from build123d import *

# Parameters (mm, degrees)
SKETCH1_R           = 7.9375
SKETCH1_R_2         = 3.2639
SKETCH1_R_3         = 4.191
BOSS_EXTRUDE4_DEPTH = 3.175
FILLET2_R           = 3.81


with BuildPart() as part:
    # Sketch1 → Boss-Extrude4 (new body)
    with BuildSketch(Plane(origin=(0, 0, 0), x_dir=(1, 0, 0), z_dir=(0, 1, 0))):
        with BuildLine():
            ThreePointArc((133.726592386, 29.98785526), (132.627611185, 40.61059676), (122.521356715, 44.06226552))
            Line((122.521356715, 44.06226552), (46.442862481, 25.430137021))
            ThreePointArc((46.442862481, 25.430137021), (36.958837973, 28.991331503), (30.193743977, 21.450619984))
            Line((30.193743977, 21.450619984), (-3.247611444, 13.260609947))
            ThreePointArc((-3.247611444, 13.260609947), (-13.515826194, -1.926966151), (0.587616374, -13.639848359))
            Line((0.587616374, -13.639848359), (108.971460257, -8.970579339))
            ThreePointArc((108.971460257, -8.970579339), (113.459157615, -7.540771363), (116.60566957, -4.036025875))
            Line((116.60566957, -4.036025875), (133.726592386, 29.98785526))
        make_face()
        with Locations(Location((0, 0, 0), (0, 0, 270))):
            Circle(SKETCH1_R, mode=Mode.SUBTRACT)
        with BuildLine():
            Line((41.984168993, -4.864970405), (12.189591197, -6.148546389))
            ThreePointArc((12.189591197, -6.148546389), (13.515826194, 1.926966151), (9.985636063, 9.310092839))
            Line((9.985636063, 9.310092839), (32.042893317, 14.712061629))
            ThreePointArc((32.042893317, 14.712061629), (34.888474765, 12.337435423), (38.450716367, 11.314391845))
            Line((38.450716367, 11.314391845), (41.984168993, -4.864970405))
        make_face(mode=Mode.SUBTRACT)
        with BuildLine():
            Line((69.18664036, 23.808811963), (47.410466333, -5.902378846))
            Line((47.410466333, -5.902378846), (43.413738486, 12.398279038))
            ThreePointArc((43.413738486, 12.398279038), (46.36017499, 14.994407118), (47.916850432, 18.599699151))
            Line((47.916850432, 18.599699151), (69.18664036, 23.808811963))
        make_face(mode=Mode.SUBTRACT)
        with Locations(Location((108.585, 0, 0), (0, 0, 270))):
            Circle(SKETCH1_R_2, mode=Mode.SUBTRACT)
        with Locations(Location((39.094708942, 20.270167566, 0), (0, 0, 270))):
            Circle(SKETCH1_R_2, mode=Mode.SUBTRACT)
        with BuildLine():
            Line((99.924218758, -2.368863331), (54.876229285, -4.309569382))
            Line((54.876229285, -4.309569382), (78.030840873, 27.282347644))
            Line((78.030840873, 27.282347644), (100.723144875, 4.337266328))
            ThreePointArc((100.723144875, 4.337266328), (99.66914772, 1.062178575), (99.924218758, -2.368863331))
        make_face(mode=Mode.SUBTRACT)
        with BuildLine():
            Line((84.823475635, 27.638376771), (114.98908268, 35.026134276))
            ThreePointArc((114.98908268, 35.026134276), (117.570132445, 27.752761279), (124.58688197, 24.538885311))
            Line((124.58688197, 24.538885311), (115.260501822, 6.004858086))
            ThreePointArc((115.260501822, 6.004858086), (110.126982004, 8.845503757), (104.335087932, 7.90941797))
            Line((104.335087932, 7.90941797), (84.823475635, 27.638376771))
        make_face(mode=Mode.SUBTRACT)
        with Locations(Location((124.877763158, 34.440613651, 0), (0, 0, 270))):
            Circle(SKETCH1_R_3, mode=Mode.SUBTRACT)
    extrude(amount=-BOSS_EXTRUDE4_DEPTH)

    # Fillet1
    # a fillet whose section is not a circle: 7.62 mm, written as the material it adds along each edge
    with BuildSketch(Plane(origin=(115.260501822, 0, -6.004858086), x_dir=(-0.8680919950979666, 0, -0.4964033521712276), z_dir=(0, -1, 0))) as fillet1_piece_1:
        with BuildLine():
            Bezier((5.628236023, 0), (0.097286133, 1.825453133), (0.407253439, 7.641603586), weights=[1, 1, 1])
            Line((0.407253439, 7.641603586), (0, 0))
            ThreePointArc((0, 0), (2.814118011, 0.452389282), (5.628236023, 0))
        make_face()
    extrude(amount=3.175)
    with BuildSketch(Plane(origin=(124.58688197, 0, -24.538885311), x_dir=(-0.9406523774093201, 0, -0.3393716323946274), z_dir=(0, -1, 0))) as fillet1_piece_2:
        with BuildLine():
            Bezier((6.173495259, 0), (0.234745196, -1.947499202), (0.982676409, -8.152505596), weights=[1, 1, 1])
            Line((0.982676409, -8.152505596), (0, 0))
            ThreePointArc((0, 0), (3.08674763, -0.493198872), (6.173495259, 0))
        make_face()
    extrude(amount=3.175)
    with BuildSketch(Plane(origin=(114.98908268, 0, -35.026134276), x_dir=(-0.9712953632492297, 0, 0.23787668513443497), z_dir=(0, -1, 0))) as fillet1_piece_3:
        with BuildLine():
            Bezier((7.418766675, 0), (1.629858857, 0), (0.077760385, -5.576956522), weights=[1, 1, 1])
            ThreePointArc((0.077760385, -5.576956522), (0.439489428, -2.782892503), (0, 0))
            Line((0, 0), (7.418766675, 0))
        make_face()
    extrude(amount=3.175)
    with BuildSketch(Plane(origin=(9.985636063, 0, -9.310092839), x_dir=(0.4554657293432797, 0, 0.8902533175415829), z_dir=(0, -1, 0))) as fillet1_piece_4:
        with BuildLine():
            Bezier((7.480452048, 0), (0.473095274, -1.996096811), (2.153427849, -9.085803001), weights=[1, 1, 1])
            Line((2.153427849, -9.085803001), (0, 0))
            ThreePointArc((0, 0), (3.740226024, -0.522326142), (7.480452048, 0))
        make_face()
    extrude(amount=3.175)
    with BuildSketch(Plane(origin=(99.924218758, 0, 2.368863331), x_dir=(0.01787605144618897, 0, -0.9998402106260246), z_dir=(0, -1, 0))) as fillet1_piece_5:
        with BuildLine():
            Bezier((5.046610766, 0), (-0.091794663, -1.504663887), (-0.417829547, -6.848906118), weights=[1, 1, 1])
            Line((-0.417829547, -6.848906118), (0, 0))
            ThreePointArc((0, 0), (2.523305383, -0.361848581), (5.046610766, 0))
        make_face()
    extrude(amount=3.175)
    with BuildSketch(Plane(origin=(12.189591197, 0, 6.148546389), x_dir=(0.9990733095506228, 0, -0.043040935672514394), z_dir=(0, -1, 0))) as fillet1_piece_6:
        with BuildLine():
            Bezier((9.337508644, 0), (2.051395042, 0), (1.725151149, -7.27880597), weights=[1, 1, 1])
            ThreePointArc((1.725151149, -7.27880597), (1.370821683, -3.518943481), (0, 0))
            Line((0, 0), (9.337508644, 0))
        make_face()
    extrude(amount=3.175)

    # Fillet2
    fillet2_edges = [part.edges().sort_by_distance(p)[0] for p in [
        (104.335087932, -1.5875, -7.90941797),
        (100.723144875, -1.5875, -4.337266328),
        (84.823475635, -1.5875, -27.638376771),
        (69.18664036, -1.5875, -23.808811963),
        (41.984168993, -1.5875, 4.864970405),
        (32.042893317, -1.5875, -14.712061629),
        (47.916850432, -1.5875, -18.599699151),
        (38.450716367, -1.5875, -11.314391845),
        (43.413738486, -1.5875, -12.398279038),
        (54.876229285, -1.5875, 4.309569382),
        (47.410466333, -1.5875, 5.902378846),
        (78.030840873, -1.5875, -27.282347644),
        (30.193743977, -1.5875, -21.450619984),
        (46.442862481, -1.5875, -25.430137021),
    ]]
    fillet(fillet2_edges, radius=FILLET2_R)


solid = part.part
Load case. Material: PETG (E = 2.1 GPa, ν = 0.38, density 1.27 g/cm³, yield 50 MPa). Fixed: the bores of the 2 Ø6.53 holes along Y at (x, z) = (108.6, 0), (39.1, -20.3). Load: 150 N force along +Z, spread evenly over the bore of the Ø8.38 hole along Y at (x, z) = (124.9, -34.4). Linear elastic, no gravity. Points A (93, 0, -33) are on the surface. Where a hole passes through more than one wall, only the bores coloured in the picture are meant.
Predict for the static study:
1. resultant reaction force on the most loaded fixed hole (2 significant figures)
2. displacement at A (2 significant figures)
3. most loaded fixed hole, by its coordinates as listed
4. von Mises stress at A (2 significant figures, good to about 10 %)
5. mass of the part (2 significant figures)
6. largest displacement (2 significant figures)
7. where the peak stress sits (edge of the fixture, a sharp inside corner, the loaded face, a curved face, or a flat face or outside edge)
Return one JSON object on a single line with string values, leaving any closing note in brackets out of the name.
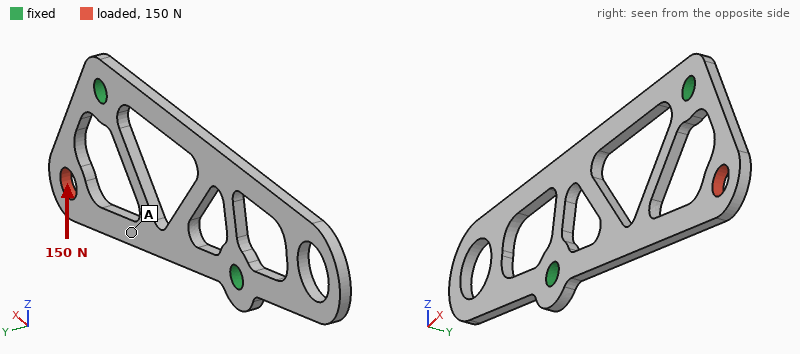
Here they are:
{"resultant reaction force on the most loaded fixed hole": "170 N", "displacement at A": "0.13 mm", "most loaded fixed hole, by its coordinates as listed": "(108.6, 0)", "von Mises stress at A": "2.5 MPa", "mass of the part": "13 g", "largest displacement": "0.34 mm", "where the peak stress sits": "a curved face"}
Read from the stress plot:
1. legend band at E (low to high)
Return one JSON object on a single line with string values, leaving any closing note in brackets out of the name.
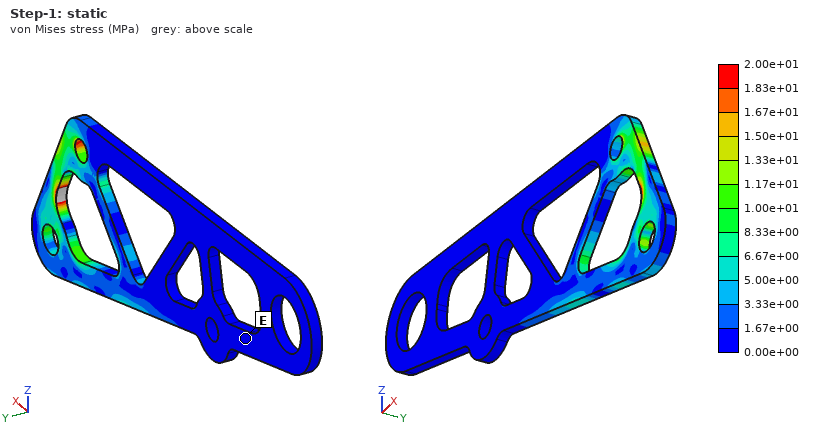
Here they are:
{"legend band at E": "0.00e+00 to 1.67e+00 MPa"}
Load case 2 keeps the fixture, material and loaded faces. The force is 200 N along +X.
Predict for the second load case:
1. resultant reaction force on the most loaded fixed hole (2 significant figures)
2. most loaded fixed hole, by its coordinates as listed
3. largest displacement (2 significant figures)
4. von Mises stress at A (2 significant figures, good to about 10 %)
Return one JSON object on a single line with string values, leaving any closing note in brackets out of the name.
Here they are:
{"resultant reaction force on the most loaded fixed hole": "130 N", "most loaded fixed hole, by its coordinates as listed": "(39.1, -20.3)", "largest displacement": "0.41 mm", "von Mises stress at A": "7.9 MPa"}
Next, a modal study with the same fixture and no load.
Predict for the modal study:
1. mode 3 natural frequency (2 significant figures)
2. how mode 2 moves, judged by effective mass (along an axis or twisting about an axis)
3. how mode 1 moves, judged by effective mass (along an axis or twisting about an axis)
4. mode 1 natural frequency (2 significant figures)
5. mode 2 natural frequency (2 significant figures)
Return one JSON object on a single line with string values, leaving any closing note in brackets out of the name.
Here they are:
{"mode 3 natural frequency": "460 Hz", "how mode 2 moves, judged by effective mass": "along Y", "how mode 1 moves, judged by effective mass": "along Y", "mode 1 natural frequency": "200 Hz", "mode 2 natural frequency": "260 Hz"}
